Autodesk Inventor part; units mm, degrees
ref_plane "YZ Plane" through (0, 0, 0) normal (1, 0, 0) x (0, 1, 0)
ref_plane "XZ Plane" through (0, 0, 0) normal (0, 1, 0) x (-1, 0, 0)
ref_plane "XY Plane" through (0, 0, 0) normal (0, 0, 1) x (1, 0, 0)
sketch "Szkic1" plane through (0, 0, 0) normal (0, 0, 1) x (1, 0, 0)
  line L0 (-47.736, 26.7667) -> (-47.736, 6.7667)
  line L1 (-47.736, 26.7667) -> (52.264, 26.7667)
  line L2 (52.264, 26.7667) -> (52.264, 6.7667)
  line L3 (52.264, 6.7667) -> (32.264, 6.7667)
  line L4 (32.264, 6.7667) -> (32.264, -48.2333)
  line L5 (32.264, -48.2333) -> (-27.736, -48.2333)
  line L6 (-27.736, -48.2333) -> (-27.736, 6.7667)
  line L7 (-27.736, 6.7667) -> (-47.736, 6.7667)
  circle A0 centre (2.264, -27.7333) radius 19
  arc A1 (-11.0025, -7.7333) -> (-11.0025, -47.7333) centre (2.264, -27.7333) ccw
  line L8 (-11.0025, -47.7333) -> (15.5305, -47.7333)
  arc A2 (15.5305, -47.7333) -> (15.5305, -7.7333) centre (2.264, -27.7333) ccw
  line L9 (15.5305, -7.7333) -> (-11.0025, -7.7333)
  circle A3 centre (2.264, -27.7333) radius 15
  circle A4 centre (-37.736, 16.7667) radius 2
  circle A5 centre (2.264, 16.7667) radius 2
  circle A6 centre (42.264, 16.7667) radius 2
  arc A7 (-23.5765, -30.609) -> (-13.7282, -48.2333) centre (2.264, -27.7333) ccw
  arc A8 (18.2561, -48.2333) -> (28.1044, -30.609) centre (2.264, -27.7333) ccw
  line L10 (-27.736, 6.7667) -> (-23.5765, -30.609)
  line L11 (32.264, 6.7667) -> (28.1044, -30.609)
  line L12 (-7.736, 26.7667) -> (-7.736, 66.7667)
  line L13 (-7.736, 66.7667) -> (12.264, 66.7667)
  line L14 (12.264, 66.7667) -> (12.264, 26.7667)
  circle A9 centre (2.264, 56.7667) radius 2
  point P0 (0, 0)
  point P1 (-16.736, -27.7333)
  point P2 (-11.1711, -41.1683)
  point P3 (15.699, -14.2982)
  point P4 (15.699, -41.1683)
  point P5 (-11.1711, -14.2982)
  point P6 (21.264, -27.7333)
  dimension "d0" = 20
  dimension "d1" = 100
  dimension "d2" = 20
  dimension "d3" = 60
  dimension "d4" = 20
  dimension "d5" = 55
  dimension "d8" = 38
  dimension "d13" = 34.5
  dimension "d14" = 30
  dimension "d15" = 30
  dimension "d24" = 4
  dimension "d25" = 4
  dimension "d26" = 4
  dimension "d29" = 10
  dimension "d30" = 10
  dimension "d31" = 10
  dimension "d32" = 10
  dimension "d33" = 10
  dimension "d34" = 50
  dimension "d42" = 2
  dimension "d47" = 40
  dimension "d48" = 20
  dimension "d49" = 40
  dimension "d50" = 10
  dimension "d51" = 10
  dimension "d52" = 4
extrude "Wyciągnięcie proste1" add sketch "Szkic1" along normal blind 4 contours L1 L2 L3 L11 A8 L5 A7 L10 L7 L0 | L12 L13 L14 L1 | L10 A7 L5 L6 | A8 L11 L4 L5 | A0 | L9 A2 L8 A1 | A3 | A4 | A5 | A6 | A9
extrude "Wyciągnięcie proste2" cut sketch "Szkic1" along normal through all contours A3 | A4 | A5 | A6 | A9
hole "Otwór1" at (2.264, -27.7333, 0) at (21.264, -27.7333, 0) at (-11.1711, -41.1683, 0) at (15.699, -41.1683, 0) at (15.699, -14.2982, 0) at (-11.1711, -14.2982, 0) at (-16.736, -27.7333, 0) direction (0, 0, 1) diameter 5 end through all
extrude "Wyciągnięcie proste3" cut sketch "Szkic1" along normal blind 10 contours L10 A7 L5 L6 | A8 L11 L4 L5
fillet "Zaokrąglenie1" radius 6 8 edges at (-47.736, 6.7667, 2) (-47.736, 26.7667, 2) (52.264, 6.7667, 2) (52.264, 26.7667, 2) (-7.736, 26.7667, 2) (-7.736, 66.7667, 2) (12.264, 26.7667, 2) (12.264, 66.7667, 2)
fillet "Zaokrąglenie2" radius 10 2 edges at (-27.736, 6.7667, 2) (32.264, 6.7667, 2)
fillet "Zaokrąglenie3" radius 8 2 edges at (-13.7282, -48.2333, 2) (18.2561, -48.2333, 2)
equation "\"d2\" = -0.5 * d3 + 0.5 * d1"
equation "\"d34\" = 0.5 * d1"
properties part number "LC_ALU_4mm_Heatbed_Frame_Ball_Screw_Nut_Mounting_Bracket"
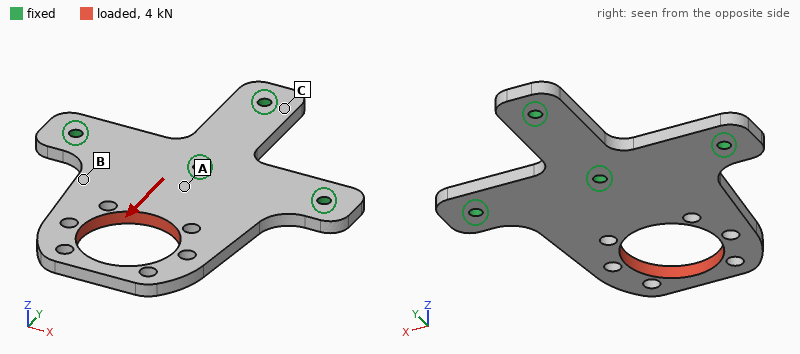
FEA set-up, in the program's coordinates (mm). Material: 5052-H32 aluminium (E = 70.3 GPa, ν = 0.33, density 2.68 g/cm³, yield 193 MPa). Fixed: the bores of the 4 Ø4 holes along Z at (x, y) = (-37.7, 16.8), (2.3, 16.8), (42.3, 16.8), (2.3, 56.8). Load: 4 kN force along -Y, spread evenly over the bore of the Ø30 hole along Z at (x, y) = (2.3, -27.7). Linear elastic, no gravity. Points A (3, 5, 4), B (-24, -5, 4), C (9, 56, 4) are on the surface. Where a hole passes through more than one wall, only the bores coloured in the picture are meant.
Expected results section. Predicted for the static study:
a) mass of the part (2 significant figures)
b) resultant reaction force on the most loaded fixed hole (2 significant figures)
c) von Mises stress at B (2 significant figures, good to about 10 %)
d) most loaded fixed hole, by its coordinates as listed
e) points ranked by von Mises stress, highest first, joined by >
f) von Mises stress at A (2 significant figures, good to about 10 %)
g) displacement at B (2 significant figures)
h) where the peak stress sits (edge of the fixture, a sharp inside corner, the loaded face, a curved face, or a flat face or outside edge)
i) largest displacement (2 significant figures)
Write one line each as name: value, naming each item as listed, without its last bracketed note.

mass of the part: 52 g
resultant reaction force on the most loaded fixed hole: 2.1 kN
von Mises stress at B: 33 MPa
most loaded fixed hole, by its coordinates as listed: (2.3, 16.8)
points ranked by von Mises stress, highest first, joined by >: B > A > C
von Mises stress at A: 18 MPa
displacement at B: 11 µm
where the peak stress sits: a curved face
largest displacement: 62 µm
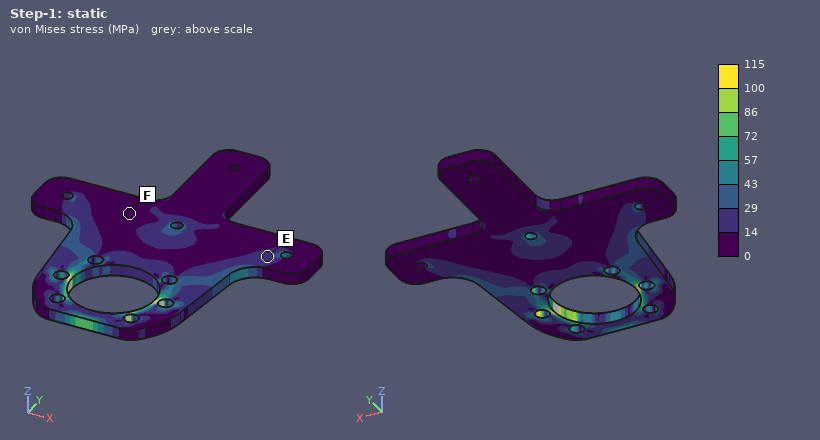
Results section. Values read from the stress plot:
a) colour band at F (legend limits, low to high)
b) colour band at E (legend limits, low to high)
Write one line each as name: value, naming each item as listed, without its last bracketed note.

colour band at F: 0 to 14 MPa
colour band at E: 14 to 29 MPa
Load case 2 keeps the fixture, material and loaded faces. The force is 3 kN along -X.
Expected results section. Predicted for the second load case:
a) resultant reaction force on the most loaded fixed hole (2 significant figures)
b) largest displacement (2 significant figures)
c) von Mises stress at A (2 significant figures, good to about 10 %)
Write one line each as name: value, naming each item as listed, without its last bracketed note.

resultant reaction force on the most loaded fixed hole: 1.9 kN
largest displacement: 0.15 mm
von Mises stress at A: 20 MPa
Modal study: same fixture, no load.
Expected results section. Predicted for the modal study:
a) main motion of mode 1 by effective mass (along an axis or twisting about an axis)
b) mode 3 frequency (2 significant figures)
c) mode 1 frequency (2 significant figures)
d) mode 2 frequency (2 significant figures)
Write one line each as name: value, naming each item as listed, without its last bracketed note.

main motion of mode 1 by effective mass: along Z
mode 3 frequency: 4000 Hz
mode 1 frequency: 1000 Hz
mode 2 frequency: 2400 Hz
